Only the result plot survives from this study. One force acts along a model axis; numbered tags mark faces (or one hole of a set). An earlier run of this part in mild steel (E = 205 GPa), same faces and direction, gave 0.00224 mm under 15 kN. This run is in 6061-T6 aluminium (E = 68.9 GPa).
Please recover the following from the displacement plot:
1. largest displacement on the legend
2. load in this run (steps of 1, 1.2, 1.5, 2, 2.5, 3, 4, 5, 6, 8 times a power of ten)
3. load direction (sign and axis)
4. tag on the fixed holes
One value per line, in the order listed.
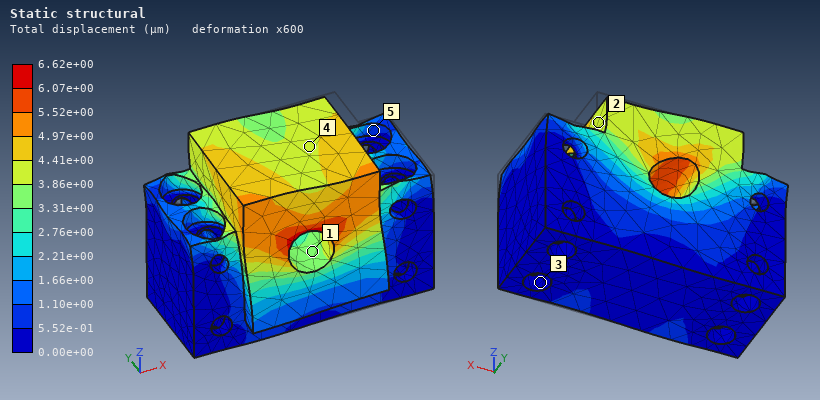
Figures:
6.62e+00 µm
15 kN
-X
3
